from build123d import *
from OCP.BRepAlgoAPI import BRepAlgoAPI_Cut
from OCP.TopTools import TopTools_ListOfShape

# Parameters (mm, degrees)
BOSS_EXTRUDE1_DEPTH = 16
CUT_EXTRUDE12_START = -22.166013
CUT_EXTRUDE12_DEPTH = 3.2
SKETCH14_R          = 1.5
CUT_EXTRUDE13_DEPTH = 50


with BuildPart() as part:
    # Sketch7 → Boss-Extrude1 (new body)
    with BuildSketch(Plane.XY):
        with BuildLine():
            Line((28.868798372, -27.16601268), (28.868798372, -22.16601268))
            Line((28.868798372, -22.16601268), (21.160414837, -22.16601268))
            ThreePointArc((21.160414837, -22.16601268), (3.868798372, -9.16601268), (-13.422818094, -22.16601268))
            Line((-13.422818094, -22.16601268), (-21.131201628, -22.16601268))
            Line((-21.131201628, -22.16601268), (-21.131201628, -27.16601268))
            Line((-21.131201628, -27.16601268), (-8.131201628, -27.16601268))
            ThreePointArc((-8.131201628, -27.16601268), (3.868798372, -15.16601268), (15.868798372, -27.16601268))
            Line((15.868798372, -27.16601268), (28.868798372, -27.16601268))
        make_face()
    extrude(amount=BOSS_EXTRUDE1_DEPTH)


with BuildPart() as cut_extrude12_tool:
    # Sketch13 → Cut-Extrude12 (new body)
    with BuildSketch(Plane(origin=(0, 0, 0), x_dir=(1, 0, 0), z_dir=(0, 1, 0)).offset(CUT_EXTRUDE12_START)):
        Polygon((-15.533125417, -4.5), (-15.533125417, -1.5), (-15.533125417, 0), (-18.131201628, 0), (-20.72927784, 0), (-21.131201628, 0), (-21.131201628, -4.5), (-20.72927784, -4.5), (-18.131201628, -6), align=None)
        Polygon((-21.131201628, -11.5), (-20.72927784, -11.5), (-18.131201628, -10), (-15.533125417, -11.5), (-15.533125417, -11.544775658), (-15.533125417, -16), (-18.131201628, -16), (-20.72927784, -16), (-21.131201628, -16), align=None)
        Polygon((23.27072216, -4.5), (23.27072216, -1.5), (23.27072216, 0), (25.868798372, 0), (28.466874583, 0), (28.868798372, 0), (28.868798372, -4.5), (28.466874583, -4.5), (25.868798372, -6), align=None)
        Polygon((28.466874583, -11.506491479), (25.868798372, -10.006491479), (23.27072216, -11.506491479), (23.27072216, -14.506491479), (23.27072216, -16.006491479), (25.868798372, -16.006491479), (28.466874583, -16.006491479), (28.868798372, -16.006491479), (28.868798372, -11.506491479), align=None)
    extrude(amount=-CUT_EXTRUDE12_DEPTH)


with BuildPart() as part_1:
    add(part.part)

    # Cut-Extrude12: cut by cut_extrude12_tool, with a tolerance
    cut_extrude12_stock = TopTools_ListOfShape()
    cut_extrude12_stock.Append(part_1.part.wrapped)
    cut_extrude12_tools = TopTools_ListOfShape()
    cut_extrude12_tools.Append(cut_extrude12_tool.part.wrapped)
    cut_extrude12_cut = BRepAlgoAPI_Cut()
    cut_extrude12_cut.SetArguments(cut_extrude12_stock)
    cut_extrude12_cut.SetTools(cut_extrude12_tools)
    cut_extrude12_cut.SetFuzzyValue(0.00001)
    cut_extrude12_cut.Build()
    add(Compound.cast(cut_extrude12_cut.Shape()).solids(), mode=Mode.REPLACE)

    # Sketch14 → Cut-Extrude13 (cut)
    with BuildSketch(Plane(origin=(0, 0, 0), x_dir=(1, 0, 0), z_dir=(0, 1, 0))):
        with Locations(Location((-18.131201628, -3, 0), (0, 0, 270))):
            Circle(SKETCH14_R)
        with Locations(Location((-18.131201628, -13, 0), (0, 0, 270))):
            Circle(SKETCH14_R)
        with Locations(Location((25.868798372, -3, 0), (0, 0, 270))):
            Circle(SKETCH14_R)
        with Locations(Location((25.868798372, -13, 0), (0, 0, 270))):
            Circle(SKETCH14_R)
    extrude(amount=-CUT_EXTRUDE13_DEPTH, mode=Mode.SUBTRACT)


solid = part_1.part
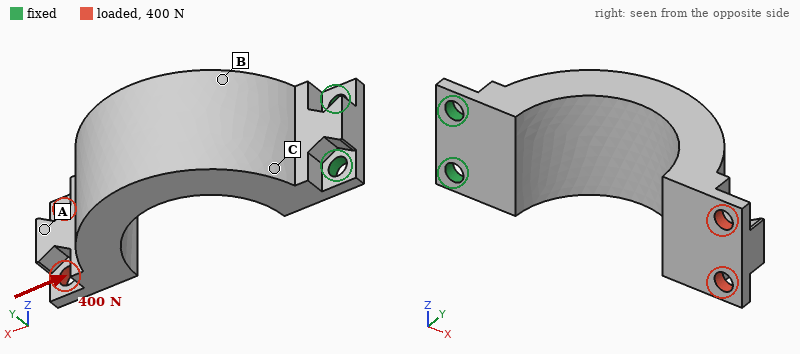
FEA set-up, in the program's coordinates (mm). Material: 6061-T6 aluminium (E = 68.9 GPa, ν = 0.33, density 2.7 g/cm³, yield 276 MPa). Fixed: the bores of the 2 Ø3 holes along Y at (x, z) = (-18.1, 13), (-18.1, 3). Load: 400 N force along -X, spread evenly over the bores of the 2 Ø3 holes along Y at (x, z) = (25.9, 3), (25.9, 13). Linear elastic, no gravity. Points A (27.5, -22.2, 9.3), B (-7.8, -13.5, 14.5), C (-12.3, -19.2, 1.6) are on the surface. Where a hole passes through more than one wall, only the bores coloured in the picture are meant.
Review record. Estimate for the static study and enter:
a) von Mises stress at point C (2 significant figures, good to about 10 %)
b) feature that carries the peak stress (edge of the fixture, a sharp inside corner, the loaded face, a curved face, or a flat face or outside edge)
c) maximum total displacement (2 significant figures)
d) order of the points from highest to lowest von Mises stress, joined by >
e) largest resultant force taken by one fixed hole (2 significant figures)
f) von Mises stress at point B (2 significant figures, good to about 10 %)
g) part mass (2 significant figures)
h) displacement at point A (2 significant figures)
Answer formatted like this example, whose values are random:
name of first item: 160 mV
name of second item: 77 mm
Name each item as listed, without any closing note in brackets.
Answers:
von Mises stress at point C: 20 MPa
feature that carries the peak stress: a curved face
maximum total displacement: 0.24 mm
order of the points from highest to lowest von Mises stress, joined by >: B > C > A
largest resultant force taken by one fixed hole: 200 N
von Mises stress at point B: 37 MPa
part mass: 14 g
displacement at point A: 0.21 mm
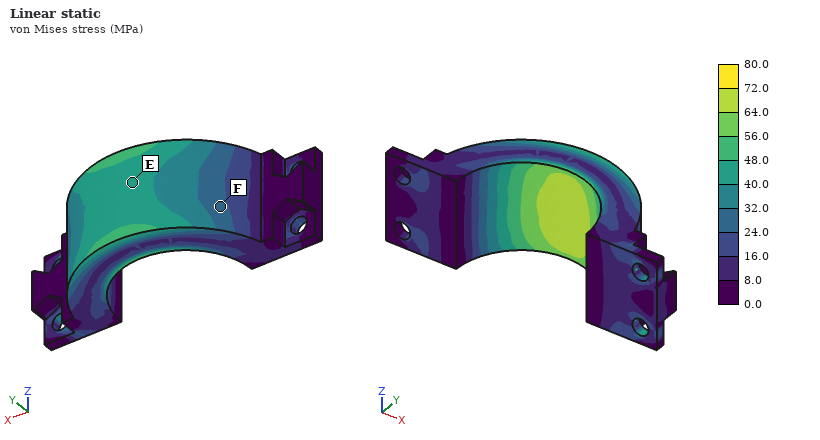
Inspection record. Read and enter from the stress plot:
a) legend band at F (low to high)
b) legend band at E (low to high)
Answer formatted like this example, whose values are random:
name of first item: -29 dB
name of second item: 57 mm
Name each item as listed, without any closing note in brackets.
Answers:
legend band at F: 24.0 to 32.0 MPa
legend band at E: 40.0 to 48.0 MPa
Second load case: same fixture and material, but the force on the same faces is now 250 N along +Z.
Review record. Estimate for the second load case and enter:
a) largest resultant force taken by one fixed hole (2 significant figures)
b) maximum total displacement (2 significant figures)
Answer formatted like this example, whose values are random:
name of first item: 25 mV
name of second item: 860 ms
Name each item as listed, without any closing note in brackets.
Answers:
largest resultant force taken by one fixed hole: 960 N
maximum total displacement: 0.30 mm
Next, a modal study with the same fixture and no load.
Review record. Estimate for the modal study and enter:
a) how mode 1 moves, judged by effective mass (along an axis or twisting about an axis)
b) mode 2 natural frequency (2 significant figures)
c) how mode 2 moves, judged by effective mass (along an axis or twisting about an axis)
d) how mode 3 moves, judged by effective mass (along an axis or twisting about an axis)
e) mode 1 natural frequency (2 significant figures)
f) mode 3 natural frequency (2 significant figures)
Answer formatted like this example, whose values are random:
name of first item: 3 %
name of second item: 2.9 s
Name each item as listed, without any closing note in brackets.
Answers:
how mode 1 moves, judged by effective mass: along Y
mode 2 natural frequency: 2800 Hz
how mode 2 moves, judged by effective mass: along Z
how mode 3 moves, judged by effective mass: along X
mode 1 natural frequency: 1000 Hz
mode 3 natural frequency: 5200 Hz
